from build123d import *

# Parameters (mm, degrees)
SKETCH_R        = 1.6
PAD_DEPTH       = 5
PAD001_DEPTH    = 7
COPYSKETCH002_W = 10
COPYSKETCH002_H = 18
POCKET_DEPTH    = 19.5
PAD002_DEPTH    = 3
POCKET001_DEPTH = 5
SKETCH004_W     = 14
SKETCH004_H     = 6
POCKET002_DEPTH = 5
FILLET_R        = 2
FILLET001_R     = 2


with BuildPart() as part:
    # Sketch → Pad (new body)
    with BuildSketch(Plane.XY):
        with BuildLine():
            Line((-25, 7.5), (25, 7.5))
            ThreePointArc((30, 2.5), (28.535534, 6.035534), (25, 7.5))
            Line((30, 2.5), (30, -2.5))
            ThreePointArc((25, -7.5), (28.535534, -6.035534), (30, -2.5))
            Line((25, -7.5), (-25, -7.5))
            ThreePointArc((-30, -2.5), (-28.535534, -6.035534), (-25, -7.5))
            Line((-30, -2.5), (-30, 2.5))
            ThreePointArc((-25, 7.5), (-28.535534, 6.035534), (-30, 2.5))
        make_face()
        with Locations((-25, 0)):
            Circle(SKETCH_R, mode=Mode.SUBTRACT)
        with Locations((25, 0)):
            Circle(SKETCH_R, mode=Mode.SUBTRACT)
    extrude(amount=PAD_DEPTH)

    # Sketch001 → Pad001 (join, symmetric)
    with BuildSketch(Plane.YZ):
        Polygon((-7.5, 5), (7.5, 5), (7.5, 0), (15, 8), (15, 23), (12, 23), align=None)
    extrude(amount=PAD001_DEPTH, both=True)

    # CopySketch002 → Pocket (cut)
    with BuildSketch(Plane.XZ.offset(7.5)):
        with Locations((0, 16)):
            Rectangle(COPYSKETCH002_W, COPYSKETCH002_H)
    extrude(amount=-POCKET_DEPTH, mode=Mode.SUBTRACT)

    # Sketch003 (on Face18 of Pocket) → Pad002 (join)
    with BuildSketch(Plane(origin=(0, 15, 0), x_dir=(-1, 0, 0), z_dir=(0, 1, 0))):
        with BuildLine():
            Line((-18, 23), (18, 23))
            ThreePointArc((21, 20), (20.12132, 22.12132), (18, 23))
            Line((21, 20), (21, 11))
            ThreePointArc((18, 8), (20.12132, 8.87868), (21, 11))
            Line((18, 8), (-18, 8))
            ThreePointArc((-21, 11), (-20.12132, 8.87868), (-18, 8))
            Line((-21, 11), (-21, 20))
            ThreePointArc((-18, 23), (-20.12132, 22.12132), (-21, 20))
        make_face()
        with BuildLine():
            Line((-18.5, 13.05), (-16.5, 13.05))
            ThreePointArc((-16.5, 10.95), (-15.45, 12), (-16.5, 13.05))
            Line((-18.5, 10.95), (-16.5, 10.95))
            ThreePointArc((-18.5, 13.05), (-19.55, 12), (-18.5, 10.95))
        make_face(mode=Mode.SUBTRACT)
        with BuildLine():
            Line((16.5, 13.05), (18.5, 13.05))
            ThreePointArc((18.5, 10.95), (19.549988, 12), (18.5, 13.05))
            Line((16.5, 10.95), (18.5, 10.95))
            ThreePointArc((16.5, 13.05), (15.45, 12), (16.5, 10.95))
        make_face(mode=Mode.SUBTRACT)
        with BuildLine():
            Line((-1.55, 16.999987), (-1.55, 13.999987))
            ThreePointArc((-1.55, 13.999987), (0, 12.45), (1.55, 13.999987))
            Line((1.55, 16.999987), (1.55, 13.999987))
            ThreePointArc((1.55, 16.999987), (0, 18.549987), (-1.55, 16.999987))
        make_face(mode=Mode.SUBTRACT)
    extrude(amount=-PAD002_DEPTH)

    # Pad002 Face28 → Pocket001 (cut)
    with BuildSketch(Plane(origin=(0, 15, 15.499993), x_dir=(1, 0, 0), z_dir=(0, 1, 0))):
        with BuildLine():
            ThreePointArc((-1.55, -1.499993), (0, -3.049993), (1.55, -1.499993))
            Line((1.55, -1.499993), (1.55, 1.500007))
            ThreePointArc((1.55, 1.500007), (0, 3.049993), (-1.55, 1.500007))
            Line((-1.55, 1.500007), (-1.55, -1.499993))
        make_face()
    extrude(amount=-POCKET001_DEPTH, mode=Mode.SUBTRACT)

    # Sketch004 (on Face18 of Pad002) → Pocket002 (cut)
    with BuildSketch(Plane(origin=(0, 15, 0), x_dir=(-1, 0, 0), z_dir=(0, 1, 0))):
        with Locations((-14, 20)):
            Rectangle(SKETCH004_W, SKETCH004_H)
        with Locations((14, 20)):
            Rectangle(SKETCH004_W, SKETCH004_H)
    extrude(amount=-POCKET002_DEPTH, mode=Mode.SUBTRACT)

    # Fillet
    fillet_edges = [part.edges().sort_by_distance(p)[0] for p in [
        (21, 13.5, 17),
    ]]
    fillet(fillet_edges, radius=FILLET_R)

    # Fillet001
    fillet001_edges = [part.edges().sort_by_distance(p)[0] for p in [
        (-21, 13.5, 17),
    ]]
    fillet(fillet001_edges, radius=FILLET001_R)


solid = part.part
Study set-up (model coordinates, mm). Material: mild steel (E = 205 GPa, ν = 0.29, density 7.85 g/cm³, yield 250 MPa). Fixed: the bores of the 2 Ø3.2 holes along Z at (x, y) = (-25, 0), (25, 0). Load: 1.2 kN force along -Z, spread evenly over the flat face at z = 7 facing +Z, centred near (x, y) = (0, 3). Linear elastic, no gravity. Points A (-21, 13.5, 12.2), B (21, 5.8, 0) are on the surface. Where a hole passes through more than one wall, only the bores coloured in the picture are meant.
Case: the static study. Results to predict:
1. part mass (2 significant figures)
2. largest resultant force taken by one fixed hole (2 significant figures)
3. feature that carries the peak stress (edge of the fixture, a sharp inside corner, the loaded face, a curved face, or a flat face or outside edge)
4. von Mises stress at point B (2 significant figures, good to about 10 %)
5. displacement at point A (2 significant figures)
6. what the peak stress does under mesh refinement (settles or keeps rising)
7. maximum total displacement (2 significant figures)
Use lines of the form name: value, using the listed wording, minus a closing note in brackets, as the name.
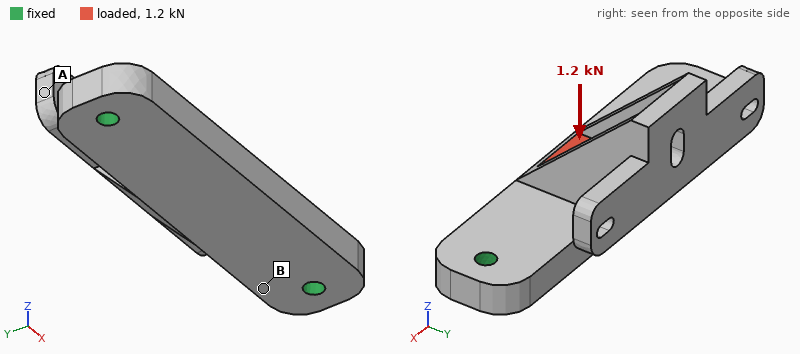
part mass: 54 g
largest resultant force taken by one fixed hole: 650 N
feature that carries the peak stress: edge of the fixture
von Mises stress at point B: 59 MPa
displacement at point A: 31 µm
what the peak stress does under mesh refinement: keeps rising
maximum total displacement: 38 µm
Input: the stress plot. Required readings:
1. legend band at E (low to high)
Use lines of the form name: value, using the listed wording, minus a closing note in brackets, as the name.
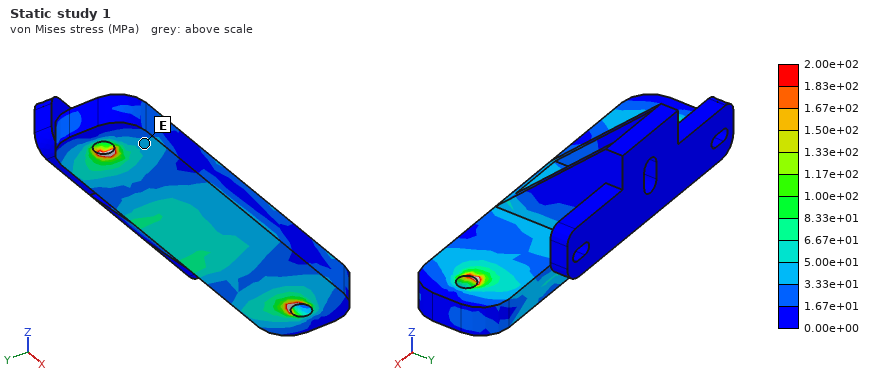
legend band at E: 3.33e+01 to 5.00e+01 MPa
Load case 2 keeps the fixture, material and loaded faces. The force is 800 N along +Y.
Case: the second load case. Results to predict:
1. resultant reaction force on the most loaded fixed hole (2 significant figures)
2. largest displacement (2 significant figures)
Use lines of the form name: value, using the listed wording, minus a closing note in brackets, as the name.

resultant reaction force on the most loaded fixed hole: 400 N
largest displacement: 26 µm
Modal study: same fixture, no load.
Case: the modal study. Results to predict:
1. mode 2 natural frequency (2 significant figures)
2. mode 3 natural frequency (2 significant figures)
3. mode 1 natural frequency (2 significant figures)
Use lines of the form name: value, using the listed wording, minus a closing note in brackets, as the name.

mode 2 natural frequency: 6700 Hz
mode 3 natural frequency: 7800 Hz
mode 1 natural frequency: 4300 Hz
